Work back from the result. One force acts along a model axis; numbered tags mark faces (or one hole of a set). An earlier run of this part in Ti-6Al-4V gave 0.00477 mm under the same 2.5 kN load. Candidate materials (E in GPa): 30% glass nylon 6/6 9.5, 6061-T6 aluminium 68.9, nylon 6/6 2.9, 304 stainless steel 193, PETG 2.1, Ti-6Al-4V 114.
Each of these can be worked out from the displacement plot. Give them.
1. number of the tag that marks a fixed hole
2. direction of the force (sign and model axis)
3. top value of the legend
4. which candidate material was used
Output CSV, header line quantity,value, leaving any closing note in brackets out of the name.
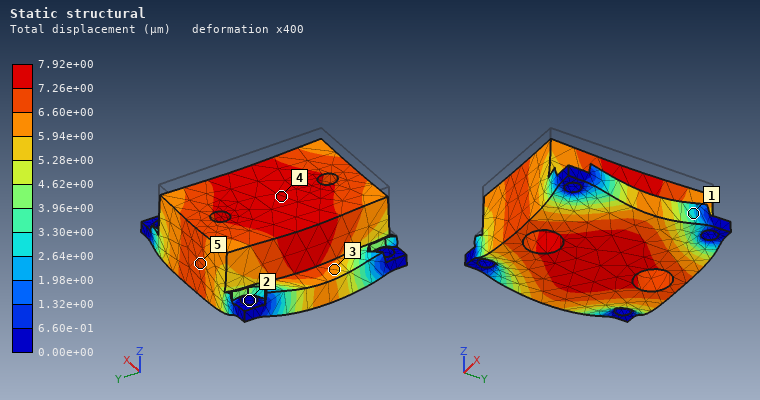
quantity,value
number of the tag that marks a fixed hole,2
direction of the force,-Z
top value of the legend,7.92e+00 µm
which candidate material was used,6061-T6 aluminium
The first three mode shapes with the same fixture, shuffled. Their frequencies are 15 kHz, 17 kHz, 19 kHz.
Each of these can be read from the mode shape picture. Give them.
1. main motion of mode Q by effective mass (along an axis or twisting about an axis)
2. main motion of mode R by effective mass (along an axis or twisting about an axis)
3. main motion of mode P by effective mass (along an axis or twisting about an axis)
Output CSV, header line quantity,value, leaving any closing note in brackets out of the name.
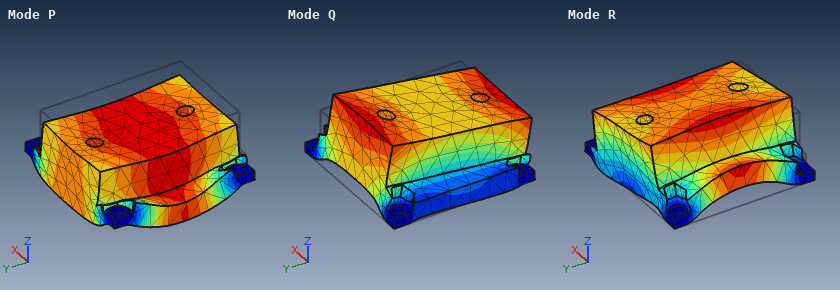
quantity,value
main motion of mode Q by effective mass,along Y
main motion of mode R by effective mass,along X
main motion of mode P by effective mass,along Z
